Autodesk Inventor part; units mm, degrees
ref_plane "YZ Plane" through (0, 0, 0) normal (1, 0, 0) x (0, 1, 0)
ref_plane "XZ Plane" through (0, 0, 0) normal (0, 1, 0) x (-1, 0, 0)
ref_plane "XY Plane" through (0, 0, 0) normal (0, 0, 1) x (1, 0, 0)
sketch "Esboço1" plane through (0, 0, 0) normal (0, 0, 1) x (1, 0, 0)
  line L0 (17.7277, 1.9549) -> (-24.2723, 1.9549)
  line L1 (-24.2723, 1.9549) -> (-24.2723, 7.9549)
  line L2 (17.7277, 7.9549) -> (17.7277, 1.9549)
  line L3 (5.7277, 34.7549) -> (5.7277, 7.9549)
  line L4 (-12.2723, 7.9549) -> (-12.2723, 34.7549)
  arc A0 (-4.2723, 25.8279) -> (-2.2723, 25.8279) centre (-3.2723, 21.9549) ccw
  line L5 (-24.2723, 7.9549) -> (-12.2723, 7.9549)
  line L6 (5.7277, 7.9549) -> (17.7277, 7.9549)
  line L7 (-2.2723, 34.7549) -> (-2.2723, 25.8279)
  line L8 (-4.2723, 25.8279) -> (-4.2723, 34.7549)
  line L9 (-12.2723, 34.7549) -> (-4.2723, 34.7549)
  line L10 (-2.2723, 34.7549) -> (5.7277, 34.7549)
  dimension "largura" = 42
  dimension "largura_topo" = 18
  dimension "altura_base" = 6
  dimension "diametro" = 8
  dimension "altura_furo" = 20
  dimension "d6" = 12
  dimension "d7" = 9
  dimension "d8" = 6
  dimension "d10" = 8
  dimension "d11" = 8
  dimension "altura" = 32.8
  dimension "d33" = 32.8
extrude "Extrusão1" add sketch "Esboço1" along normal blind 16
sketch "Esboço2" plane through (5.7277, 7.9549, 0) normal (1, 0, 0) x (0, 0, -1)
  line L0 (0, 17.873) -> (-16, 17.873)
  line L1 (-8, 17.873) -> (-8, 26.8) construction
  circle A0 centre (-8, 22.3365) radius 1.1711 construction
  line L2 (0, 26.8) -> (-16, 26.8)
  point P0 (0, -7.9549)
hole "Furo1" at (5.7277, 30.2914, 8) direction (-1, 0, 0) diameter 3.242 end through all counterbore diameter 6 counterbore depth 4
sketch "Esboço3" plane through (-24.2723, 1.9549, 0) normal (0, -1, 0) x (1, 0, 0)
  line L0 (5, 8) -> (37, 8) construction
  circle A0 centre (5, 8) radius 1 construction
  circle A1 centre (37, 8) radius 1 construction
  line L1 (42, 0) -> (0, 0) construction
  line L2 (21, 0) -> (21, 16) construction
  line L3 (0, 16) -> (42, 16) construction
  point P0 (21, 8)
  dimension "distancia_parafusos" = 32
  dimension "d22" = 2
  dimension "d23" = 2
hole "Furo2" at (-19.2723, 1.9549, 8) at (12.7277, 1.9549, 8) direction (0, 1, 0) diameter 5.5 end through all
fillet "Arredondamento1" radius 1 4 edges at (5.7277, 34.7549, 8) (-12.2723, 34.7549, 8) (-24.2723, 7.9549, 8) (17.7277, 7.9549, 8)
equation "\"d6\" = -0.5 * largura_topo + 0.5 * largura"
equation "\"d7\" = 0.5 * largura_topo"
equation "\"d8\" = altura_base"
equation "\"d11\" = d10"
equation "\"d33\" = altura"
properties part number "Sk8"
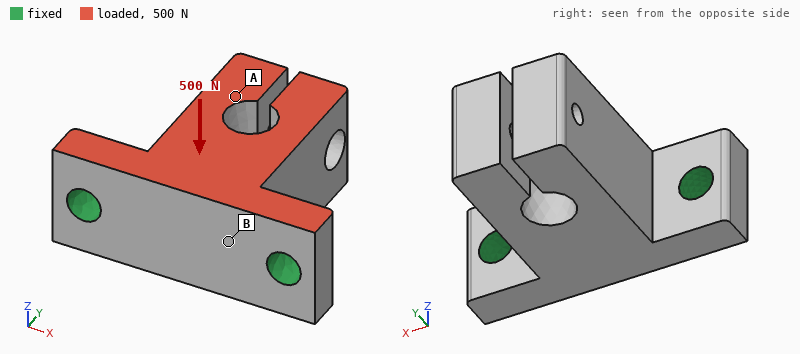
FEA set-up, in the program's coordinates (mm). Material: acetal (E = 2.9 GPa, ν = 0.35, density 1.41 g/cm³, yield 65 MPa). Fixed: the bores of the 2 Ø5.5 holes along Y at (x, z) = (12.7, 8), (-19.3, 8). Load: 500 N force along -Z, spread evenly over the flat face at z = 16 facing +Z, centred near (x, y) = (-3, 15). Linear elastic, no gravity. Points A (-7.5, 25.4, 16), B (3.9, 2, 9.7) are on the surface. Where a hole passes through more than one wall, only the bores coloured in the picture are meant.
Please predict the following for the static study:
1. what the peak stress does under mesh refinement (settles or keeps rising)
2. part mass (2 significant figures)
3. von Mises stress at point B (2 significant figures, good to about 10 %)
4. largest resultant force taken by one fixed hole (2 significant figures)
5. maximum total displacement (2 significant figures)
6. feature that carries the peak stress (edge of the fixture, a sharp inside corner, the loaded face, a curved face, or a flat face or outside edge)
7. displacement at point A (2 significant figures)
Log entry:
keeps rising
14 g
7.0 MPa
250 N
0.58 mm
edge of the fixture
0.42 mm
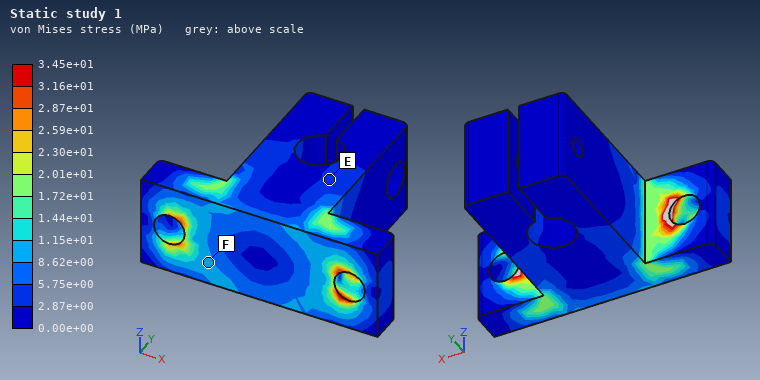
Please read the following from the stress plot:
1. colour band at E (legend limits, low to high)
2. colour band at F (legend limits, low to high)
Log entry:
2.87e+00 to 5.75e+00 MPa
8.62e+00 to 1.15e+01 MPa
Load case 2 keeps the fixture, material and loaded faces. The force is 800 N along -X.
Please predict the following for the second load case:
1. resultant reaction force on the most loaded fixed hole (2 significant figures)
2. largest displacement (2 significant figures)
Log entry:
550 N
0.51 mm
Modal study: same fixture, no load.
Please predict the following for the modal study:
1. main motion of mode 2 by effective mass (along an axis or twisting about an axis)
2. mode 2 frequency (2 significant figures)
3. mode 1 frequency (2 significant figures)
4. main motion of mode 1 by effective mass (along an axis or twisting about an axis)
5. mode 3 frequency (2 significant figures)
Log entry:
along X
2400 Hz
1500 Hz
along Z
2900 Hz
